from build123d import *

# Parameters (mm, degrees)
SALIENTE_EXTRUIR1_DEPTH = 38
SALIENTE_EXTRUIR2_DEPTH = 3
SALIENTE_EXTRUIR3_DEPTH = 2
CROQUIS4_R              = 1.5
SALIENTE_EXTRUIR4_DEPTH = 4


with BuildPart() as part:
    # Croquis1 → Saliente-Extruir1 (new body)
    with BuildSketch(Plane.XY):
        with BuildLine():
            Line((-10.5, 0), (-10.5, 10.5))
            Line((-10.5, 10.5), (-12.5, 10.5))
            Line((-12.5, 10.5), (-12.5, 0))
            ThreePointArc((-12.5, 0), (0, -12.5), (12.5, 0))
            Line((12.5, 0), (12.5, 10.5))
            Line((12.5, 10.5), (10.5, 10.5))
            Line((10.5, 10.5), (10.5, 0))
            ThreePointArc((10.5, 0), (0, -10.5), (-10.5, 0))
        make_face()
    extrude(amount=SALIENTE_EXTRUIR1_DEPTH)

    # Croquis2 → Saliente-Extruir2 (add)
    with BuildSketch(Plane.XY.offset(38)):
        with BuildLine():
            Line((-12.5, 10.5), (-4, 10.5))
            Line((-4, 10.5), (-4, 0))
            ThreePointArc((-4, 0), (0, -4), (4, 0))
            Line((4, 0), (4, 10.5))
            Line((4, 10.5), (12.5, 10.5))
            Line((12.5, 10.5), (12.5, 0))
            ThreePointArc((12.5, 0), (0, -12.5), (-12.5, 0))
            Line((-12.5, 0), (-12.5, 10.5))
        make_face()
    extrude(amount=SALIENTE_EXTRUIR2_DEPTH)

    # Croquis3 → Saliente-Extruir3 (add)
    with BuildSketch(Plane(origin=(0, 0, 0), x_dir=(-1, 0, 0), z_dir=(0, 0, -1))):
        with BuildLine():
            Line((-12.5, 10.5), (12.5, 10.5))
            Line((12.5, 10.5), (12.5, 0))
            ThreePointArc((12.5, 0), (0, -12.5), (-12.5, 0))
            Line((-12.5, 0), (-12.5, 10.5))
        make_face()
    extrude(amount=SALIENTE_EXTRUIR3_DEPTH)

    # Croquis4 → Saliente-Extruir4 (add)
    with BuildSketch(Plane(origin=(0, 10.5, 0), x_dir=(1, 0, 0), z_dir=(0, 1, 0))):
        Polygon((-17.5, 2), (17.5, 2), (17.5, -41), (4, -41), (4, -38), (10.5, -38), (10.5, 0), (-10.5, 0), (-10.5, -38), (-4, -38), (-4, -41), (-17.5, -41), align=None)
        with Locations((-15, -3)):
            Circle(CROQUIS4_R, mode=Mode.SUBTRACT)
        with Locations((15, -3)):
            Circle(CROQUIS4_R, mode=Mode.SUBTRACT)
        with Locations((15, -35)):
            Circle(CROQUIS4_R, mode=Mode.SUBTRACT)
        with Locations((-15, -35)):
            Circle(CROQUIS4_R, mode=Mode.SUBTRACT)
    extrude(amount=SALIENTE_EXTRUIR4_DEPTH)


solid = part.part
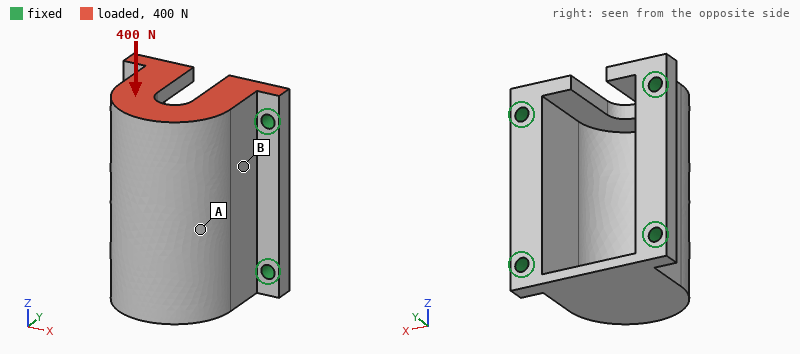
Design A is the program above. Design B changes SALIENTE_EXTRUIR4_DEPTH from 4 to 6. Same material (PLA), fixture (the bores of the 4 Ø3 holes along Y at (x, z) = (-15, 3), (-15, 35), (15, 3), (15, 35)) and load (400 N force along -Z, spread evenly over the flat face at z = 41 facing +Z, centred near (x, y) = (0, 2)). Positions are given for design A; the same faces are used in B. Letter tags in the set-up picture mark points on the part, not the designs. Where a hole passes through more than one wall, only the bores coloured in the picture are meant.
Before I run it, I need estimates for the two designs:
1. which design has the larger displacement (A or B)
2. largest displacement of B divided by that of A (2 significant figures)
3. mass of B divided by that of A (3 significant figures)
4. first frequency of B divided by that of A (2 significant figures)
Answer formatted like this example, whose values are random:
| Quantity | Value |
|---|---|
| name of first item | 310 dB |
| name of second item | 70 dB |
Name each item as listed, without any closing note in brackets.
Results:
| Quantity | Value |
|---|---|
| which design has the larger displacement | A |
| largest displacement of B divided by that of A | 0.84 |
| mass of B divided by that of A | 1.14 |
| first frequency of B divided by that of A | 1.0 |
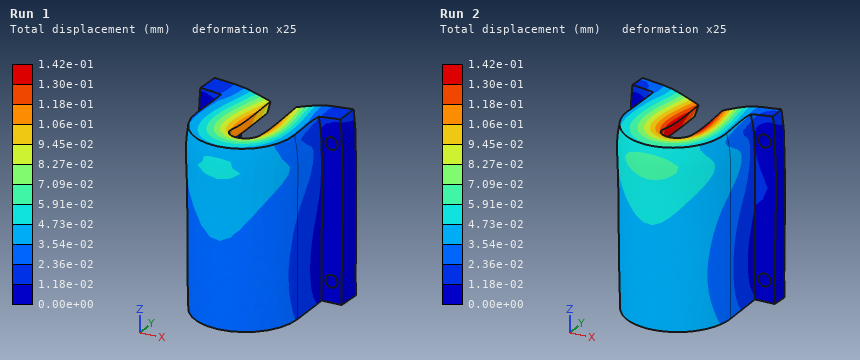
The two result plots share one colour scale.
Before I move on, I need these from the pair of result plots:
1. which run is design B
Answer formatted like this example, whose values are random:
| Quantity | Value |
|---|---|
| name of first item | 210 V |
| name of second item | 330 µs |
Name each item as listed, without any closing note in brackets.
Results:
| Quantity | Value |
|---|---|
| which run is design B | Run 1 |
